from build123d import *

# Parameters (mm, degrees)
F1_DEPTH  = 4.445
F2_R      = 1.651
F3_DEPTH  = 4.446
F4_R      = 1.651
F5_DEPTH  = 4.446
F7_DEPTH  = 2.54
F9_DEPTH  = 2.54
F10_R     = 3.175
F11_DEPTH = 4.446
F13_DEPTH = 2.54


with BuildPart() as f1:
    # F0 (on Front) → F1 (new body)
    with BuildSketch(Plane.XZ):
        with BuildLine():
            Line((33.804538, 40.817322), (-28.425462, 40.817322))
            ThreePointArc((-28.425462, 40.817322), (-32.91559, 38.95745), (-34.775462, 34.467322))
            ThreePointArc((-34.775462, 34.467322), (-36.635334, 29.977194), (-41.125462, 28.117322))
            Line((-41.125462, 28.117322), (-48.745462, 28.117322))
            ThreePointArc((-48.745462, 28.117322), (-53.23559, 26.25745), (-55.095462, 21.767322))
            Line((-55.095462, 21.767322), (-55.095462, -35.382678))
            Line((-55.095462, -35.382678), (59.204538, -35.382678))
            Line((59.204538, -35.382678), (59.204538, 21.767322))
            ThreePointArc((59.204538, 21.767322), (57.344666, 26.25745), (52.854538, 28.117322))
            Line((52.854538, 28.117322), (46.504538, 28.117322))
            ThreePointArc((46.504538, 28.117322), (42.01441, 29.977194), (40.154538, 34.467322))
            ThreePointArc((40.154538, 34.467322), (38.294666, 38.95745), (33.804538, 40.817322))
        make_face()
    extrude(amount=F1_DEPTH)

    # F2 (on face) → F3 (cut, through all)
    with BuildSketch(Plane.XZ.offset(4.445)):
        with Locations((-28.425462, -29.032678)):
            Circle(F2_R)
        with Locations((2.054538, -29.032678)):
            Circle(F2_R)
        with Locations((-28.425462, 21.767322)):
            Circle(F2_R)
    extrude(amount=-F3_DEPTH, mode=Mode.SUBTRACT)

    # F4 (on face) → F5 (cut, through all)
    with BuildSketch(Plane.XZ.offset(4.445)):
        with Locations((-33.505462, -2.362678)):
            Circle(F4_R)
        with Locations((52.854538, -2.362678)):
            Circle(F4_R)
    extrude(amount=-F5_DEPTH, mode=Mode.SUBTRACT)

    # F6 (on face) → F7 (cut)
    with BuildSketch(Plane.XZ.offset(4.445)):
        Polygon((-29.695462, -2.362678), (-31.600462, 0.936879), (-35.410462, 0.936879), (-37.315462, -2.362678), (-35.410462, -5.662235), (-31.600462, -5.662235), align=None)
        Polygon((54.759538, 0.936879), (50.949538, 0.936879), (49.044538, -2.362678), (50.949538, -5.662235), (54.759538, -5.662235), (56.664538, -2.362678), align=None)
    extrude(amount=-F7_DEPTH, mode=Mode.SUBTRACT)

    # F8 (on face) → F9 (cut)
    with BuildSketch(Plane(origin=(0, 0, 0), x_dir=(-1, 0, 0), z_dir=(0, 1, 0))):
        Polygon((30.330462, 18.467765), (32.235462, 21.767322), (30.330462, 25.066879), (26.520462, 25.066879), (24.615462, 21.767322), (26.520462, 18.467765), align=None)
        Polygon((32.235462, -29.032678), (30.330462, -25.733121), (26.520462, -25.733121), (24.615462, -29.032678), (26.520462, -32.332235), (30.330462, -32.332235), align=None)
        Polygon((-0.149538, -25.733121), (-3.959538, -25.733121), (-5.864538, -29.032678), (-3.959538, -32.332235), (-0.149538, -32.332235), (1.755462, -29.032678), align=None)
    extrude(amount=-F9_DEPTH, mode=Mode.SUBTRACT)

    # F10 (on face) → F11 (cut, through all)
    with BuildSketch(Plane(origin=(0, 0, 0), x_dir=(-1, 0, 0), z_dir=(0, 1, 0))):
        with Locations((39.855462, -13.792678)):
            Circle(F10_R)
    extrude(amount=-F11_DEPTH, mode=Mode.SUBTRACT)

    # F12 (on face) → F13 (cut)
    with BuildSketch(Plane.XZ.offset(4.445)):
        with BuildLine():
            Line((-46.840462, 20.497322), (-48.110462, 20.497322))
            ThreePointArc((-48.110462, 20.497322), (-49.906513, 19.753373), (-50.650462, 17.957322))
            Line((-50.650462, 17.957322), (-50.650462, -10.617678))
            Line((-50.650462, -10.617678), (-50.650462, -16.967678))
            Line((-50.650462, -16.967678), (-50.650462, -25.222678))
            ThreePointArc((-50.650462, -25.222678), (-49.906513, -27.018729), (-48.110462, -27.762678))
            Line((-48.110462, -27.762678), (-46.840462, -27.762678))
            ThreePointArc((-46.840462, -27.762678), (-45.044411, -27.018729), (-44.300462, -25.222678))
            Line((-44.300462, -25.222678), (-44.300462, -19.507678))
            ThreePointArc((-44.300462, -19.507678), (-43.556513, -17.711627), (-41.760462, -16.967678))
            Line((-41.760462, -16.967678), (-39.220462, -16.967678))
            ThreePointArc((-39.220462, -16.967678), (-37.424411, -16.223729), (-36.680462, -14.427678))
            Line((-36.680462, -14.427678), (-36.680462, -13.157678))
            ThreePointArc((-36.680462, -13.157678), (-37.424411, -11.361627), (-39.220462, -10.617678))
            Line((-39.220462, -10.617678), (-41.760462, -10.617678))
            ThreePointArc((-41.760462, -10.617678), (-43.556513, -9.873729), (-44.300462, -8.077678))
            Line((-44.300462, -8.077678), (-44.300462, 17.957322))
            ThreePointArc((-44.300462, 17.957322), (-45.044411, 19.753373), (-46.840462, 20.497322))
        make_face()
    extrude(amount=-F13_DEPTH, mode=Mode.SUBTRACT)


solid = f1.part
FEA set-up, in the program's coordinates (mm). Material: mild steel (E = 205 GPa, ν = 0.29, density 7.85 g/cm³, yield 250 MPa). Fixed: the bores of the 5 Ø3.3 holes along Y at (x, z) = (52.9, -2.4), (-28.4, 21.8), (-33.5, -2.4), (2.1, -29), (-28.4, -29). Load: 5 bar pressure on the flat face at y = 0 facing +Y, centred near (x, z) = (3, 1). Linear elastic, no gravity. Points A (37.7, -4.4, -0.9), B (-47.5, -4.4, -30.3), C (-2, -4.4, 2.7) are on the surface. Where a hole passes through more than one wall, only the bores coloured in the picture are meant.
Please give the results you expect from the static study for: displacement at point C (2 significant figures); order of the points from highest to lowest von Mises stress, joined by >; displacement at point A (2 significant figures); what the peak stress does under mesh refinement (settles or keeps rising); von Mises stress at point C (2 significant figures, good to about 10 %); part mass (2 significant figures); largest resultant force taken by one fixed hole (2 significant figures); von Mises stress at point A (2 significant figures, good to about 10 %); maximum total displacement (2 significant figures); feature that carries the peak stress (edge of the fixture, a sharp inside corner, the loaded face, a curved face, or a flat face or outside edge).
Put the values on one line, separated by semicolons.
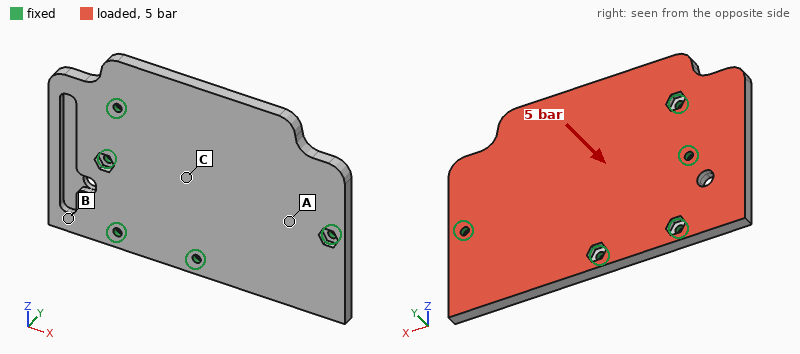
0.049 mm; A > C > B; 0.041 mm; keeps rising; 43 MPa; 270 g; 1.5 kN; 76 MPa; 0.20 mm; edge of the fixture
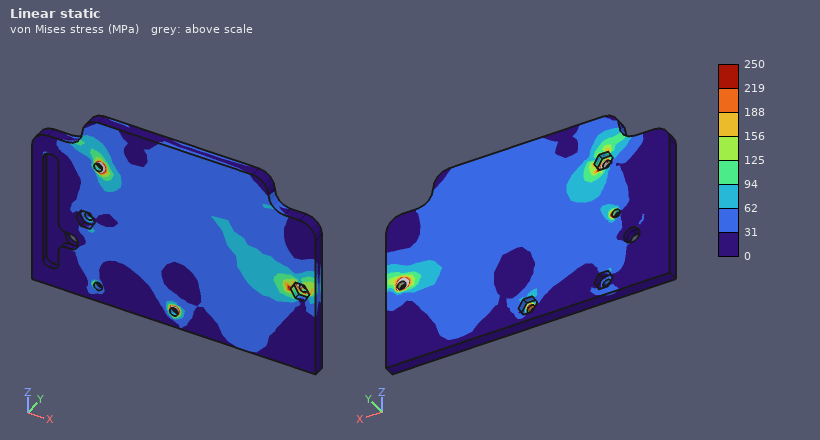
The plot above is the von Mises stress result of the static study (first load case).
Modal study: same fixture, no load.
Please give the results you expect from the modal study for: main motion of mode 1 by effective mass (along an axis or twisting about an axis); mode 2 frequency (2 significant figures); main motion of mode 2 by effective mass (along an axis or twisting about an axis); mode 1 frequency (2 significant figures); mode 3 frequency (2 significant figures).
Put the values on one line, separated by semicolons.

along Y; 3200 Hz; along Y; 1700 Hz; 4300 Hz
